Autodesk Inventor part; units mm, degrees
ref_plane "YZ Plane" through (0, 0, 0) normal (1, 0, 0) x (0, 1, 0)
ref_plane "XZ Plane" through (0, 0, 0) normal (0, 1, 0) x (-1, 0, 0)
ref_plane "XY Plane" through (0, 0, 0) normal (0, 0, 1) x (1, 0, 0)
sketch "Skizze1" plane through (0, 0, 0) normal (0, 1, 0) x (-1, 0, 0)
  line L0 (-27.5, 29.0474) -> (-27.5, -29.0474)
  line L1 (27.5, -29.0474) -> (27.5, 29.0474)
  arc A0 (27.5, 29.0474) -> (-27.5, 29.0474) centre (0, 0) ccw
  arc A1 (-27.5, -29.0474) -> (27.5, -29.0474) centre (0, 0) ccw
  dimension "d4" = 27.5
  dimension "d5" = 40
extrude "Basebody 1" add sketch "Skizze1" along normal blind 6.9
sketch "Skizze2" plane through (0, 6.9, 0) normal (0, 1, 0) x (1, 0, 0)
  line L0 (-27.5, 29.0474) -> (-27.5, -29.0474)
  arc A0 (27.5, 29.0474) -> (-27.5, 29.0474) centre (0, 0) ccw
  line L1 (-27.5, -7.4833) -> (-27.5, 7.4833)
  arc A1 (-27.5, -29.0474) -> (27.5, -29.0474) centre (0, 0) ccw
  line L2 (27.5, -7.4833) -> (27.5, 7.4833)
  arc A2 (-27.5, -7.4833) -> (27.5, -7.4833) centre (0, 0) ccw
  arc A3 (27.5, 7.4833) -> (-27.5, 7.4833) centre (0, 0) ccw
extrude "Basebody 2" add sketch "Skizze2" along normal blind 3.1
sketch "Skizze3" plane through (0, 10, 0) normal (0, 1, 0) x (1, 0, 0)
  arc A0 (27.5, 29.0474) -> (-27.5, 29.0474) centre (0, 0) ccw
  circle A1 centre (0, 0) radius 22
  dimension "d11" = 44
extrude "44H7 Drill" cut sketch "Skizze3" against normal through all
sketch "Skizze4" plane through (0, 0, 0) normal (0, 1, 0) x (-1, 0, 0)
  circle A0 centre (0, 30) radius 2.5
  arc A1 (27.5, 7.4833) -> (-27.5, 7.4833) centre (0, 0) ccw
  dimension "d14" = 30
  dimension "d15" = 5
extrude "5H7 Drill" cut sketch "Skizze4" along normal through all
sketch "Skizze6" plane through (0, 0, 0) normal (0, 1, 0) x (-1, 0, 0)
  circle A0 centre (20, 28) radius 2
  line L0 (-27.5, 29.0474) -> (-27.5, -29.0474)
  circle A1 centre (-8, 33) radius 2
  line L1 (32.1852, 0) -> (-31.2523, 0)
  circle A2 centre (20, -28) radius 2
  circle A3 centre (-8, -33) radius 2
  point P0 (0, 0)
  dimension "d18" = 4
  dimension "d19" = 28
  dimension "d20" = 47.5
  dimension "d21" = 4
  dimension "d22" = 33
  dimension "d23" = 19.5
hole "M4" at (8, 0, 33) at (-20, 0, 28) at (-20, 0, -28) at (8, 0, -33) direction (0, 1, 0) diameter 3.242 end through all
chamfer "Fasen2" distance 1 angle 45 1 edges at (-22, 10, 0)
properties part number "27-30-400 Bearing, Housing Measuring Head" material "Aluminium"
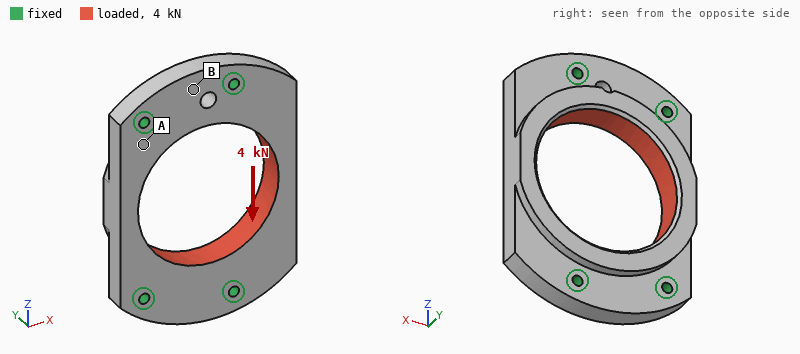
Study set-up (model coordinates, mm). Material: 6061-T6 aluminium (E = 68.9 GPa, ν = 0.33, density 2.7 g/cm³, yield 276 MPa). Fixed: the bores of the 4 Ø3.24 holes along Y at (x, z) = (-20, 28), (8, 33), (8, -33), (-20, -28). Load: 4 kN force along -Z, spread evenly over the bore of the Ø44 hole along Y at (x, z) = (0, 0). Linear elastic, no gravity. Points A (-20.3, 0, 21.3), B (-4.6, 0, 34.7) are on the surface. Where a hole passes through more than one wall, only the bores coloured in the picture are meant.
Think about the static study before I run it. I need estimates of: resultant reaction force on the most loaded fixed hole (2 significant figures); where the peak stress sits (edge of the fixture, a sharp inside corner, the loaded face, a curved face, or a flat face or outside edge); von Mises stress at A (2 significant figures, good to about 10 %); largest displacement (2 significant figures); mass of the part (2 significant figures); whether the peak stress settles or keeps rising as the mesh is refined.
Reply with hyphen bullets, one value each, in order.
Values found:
- 1.3 kN
- edge of the fixture
- 8.5 MPa
- 8.5 µm
- 54 g
- keeps rising
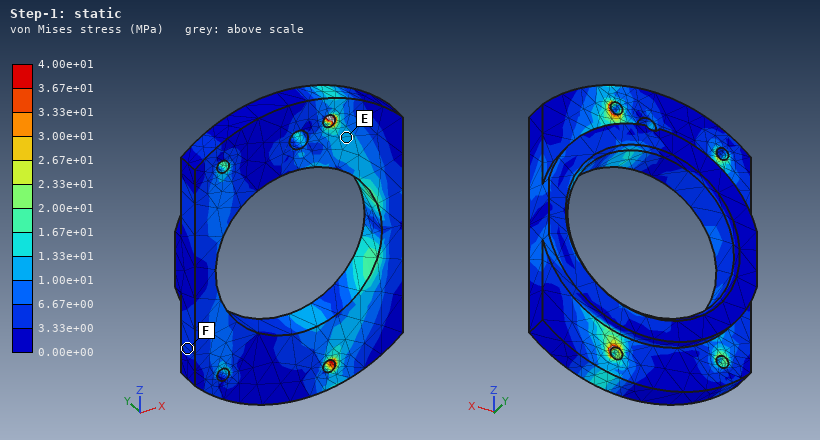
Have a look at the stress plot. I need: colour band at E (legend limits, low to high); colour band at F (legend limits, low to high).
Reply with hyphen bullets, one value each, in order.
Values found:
- 1.00e+01 to 1.33e+01 MPa
- 3.33e+00 to 6.67e+00 MPa
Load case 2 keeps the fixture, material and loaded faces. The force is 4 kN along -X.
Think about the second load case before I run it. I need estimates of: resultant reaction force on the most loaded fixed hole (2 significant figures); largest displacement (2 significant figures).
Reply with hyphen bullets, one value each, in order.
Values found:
- 1.1 kN
- 14 µm
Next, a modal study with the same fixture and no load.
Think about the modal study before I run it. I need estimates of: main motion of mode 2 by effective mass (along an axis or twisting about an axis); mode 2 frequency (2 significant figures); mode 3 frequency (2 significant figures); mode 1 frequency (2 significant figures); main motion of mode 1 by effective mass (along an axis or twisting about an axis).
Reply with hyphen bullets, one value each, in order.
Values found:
- along Y
- 13 kHz
- 14 kHz
- 6800 Hz
- along Y
